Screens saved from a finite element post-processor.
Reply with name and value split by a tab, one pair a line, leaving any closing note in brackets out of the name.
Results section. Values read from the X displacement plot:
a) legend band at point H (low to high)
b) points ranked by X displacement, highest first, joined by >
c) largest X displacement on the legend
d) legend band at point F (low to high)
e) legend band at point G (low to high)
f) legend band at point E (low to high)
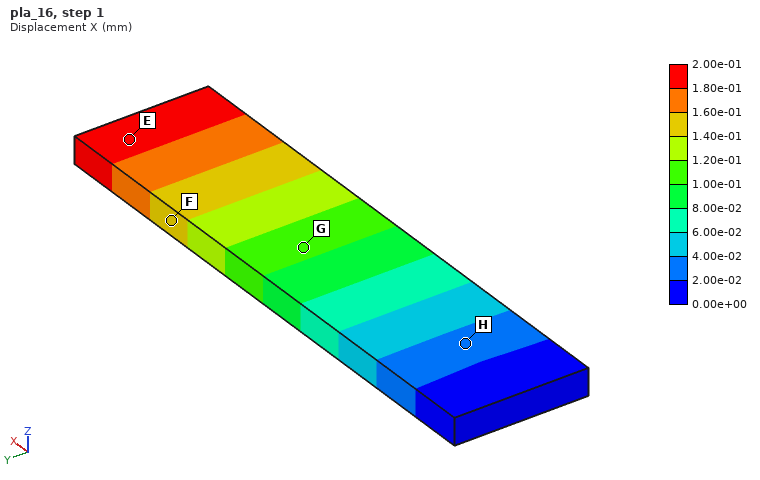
legend band at point H	2.00e-02 to 4.00e-02 mm
points ranked by X displacement, highest first, joined by >	E > F > G > H
largest X displacement on the legend	2.00e-01 mm
legend band at point F	1.40e-01 to 1.60e-01 mm
legend band at point G	1.00e-01 to 1.20e-01 mm
legend band at point E	1.80e-01 to 2.00e-01 mm
